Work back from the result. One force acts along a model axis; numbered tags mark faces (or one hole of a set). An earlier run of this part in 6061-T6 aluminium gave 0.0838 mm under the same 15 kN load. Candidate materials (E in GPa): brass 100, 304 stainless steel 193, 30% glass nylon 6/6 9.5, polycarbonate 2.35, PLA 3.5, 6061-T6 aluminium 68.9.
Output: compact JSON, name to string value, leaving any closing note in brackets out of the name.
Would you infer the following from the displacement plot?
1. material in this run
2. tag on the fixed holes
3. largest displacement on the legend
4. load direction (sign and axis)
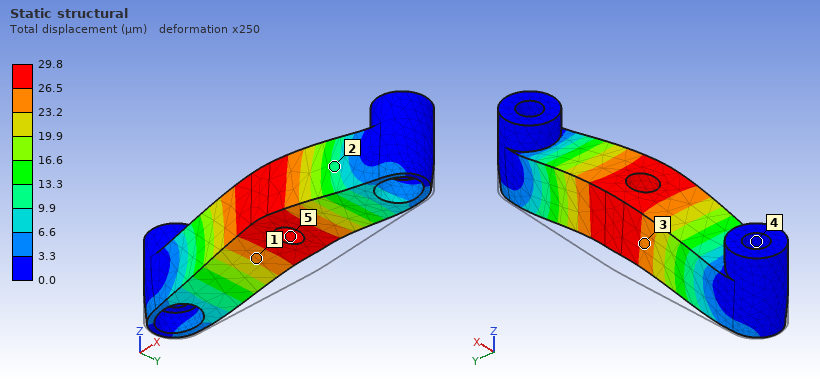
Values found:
{"material in this run": "304 stainless steel", "tag on the fixed holes": "4", "largest displacement on the legend": "29.8 µm", "load direction": "+Z"}
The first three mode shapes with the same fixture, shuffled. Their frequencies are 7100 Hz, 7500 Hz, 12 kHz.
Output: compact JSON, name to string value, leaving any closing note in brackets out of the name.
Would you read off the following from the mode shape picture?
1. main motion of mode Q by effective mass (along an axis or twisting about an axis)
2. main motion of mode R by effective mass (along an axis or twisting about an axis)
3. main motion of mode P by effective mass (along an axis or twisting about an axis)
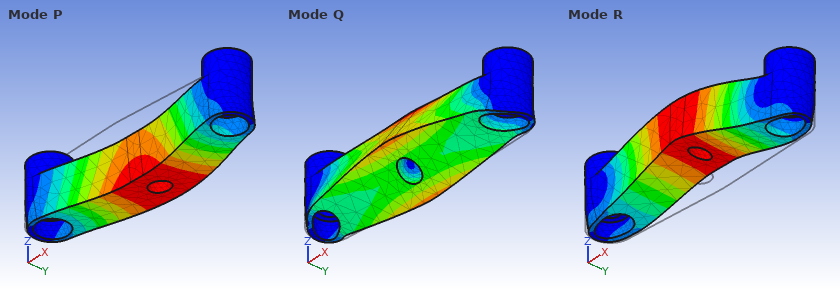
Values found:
{"main motion of mode Q by effective mass": "twisting about X", "main motion of mode R by effective mass": "along Z", "main motion of mode P by effective mass": "along Y"}
